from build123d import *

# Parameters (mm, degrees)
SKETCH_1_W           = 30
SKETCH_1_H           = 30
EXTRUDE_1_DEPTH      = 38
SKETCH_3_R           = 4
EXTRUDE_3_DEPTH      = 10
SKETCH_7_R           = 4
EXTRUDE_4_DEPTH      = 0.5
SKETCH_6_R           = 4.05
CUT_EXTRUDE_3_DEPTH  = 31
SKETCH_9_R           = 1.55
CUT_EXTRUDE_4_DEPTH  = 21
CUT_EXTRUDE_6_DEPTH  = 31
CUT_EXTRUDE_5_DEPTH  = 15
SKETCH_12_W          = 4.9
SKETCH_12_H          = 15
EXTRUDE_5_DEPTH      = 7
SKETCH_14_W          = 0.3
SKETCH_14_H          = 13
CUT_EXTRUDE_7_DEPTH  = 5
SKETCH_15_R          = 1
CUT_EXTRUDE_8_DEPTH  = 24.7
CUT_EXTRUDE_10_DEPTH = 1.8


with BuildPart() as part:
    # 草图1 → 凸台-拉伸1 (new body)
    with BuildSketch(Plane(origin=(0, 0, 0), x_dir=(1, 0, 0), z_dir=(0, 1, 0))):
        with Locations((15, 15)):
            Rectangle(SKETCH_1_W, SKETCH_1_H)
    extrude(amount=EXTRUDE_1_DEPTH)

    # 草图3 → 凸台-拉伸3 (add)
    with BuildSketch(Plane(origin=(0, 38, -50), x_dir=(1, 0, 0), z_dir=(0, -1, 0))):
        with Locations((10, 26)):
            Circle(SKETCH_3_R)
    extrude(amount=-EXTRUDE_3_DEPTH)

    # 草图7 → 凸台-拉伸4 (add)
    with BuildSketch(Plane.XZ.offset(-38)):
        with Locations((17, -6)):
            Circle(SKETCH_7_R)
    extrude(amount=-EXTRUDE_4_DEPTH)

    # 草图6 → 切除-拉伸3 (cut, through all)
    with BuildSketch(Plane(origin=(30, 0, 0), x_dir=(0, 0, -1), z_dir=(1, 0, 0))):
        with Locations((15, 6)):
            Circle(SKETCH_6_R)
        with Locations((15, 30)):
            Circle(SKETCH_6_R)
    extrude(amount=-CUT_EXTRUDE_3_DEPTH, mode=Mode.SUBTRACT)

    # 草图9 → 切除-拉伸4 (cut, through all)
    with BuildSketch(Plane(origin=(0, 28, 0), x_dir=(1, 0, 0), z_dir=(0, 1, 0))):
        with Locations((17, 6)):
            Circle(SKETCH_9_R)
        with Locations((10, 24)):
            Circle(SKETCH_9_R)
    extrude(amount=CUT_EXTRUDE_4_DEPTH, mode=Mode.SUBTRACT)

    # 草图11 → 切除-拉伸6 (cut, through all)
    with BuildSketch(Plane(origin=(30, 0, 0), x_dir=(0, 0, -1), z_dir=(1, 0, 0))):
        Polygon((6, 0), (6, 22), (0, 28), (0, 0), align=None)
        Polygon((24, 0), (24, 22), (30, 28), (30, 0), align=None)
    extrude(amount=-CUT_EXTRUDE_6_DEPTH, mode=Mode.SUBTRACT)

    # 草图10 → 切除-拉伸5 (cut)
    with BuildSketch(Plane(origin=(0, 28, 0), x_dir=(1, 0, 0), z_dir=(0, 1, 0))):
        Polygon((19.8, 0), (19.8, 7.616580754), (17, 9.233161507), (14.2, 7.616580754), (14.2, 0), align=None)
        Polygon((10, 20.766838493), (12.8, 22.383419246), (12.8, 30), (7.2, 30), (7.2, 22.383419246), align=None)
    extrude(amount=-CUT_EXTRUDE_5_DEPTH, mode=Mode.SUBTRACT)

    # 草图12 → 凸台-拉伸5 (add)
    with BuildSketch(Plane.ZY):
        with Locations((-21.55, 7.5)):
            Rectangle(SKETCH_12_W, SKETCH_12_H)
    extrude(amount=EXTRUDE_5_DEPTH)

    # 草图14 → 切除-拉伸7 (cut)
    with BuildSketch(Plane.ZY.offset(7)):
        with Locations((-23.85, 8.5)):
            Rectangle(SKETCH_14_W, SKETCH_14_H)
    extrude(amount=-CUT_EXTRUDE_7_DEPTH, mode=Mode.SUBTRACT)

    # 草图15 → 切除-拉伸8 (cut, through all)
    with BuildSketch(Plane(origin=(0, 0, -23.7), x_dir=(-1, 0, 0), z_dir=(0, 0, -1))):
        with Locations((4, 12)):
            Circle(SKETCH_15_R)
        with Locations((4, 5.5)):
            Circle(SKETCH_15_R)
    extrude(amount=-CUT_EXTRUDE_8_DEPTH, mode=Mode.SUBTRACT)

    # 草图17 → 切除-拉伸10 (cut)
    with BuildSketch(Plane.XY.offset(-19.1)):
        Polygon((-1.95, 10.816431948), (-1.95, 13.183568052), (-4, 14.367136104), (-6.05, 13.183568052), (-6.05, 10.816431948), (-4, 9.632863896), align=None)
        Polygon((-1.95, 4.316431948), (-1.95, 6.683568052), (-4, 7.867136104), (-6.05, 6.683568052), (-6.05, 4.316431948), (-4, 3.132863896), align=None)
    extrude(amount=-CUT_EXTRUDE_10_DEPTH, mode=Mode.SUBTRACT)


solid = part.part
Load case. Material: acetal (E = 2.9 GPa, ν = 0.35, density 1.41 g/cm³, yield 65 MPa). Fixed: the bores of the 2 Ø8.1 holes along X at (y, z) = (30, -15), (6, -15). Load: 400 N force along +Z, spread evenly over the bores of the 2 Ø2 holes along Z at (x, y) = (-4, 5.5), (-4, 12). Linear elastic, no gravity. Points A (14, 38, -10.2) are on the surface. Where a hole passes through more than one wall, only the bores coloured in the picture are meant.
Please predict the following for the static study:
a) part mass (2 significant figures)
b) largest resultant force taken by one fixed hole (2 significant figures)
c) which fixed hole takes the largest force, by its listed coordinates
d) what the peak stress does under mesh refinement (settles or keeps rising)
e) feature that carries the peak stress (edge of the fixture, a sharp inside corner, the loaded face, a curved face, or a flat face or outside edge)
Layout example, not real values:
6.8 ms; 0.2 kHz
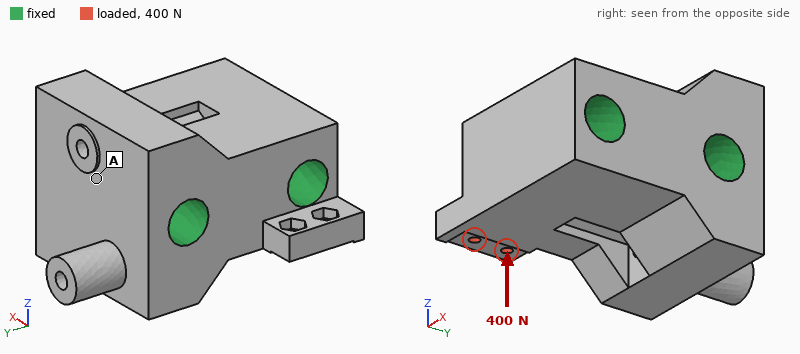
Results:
31 g; 370 N; (6, -15); keeps rising; edge of the fixture
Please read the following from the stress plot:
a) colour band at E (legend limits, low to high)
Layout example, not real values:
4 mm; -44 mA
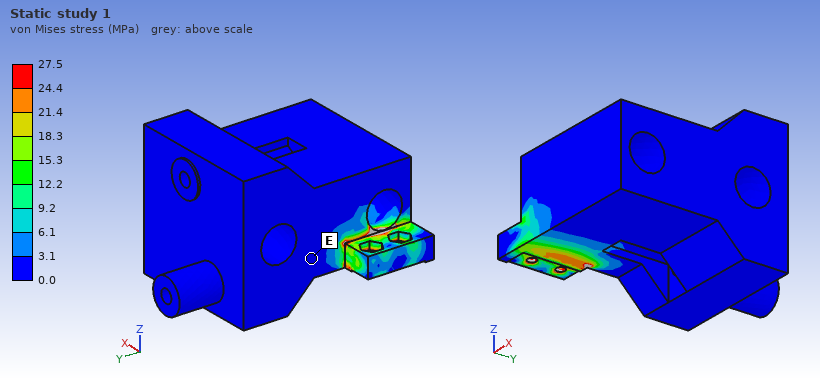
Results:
0.0 to 3.1 MPa
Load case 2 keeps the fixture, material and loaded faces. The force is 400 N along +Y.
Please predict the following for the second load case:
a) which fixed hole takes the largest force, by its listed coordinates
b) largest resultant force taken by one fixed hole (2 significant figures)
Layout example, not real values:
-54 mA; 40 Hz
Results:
(6, -15); 310 N
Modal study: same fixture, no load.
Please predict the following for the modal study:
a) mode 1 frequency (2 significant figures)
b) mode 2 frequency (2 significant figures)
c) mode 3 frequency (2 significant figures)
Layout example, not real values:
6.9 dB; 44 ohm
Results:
8800 Hz; 9400 Hz; 12 kHz
